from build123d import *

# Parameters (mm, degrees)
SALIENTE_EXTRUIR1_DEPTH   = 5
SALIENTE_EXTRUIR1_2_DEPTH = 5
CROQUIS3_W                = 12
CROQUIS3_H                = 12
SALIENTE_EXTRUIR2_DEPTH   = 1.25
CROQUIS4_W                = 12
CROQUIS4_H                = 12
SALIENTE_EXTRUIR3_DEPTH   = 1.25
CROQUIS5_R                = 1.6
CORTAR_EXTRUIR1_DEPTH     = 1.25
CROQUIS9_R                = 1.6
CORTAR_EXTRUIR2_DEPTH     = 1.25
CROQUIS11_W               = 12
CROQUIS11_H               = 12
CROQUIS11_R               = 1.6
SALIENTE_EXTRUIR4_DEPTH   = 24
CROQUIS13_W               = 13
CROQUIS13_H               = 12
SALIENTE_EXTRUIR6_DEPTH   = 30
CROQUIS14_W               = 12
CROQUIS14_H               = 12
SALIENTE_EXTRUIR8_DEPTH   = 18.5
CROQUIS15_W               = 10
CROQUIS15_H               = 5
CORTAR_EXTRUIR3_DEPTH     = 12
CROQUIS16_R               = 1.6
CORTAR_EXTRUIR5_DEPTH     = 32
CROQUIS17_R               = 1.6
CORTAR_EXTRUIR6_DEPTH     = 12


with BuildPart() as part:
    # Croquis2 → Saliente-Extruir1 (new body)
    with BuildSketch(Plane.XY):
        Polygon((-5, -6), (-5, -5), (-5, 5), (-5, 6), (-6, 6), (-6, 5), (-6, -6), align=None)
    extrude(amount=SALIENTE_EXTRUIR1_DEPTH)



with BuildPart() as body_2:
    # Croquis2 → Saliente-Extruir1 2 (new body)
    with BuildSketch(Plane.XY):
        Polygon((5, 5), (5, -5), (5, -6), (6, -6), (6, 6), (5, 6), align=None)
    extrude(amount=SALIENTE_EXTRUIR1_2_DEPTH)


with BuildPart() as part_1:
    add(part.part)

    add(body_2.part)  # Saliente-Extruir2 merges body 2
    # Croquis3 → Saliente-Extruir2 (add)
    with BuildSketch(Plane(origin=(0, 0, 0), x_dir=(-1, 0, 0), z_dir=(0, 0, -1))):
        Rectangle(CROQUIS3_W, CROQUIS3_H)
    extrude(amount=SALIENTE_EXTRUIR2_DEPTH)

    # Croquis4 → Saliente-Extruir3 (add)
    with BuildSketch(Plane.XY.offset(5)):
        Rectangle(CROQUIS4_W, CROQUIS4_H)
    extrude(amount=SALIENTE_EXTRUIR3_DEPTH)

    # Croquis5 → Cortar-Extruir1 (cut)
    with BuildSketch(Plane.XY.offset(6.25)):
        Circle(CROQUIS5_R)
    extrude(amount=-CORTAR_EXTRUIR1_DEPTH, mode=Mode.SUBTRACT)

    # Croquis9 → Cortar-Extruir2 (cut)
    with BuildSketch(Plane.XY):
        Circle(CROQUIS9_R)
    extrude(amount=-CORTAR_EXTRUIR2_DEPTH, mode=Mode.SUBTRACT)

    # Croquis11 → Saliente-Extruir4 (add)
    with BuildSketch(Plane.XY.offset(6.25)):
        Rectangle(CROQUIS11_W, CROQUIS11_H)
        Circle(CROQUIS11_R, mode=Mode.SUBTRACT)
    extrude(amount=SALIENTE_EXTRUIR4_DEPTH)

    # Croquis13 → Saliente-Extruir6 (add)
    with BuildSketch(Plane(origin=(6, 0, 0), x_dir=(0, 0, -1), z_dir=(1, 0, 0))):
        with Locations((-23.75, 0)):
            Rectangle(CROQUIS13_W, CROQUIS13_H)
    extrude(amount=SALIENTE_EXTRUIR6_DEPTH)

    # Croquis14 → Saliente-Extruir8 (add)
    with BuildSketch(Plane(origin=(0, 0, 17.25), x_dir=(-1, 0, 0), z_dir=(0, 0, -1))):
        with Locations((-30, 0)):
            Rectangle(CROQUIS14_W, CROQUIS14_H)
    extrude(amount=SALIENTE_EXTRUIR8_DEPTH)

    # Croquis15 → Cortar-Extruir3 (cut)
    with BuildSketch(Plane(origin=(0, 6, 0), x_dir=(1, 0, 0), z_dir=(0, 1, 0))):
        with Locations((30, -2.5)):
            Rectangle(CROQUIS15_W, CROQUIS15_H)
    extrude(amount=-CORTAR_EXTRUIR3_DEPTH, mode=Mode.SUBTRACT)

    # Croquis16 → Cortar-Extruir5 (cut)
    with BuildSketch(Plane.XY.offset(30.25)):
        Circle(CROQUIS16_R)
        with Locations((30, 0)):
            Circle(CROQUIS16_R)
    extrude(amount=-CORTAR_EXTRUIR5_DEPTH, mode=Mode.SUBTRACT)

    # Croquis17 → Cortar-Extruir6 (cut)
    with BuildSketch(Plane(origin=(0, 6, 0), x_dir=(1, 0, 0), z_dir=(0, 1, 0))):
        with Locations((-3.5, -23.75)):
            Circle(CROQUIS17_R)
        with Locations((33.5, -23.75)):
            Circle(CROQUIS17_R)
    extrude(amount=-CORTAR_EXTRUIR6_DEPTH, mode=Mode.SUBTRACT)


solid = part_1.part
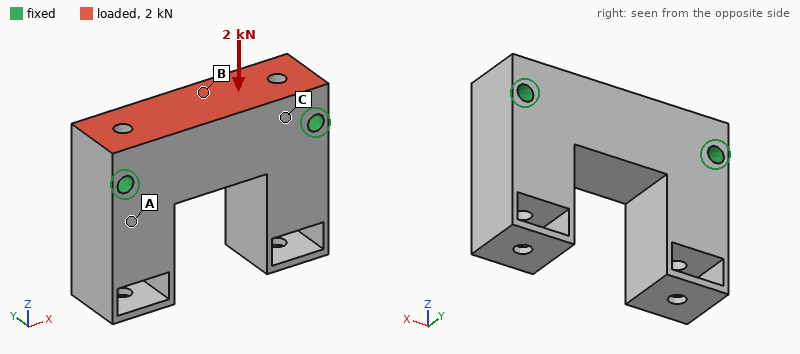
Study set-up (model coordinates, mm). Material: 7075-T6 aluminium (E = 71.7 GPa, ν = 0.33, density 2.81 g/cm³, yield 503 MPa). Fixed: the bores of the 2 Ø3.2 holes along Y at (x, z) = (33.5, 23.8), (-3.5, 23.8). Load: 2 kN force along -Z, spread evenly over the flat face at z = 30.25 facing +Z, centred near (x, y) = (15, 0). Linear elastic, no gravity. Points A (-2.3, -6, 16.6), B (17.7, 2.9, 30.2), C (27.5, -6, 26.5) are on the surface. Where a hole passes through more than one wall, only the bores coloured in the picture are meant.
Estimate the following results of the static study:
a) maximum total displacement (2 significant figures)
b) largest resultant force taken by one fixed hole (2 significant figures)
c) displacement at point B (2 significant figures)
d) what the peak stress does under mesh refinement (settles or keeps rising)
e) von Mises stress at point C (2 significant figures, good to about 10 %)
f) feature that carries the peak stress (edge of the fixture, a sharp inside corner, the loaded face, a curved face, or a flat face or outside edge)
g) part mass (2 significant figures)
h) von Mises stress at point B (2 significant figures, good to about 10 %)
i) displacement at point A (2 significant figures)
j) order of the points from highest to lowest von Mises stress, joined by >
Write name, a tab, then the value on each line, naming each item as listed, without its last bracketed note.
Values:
maximum total displacement	11 µm
largest resultant force taken by one fixed hole	1.0 kN
displacement at point B	6.1 µm
what the peak stress does under mesh refinement	keeps rising
von Mises stress at point C	11 MPa
feature that carries the peak stress	edge of the fixture
part mass	28 g
von Mises stress at point B	15 MPa
displacement at point A	2.4 µm
order of the points from highest to lowest von Mises stress, joined by >	B > C > A
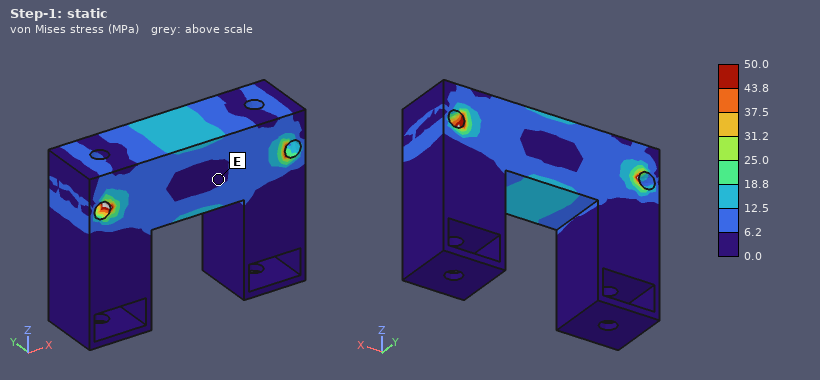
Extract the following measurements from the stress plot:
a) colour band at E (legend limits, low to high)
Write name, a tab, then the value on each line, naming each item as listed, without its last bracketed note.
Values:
colour band at E	0.0 to 6.2 MPa
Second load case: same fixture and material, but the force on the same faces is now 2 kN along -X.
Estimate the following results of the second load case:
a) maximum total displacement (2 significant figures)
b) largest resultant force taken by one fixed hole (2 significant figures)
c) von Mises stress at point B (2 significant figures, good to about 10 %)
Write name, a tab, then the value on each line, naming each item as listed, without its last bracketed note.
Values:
maximum total displacement	2.3 µm
largest resultant force taken by one fixed hole	1.0 kN
von Mises stress at point B	7.1 MPa
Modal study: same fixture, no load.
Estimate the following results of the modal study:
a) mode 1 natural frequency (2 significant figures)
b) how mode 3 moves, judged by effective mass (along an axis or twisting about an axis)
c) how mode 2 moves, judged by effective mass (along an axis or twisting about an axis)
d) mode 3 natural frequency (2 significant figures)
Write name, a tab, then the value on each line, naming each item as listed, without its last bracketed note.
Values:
mode 1 natural frequency	12 kHz
how mode 3 moves, judged by effective mass	along Y
how mode 2 moves, judged by effective mass	along X
mode 3 natural frequency	15 kHz
